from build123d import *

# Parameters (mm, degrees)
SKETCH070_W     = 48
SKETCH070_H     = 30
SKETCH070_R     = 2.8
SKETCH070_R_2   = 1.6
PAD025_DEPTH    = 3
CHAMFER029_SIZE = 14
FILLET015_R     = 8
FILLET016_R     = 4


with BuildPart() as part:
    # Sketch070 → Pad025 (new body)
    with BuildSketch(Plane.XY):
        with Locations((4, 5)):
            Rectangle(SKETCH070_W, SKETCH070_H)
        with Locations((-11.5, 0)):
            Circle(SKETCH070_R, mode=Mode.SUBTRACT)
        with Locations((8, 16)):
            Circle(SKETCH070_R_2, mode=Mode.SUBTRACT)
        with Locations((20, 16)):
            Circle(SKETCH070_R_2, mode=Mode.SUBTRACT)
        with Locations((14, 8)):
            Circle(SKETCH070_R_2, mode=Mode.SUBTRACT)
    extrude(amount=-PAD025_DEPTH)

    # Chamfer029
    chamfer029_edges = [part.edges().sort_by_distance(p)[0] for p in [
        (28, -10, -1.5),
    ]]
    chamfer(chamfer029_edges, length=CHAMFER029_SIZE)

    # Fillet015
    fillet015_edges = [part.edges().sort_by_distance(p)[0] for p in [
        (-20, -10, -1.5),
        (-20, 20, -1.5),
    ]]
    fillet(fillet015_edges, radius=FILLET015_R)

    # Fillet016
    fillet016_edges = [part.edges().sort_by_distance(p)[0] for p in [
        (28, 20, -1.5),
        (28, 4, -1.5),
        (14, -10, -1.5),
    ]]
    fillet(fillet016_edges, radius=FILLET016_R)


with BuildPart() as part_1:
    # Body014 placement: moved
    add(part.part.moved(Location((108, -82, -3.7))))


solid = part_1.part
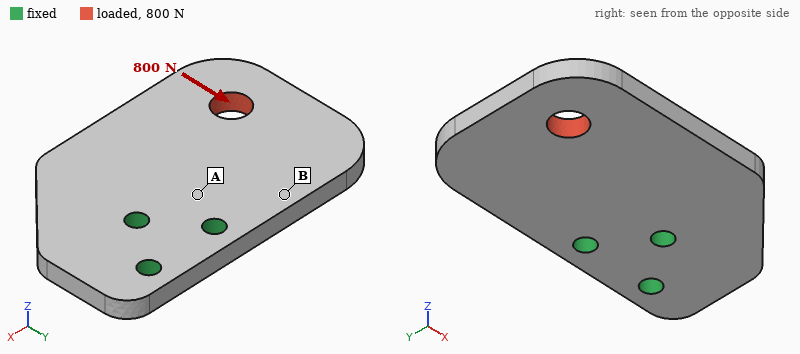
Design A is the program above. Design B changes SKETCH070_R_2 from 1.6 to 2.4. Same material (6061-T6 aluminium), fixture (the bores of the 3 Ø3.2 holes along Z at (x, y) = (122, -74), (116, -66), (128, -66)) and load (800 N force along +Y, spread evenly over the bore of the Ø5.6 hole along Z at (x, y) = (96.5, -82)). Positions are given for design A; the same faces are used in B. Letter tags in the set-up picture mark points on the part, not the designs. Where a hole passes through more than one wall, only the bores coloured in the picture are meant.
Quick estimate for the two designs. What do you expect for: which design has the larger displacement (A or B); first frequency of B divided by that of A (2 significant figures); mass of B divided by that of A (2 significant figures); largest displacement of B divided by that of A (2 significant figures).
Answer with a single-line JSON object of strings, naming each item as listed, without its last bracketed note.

{"which design has the larger displacement": "A", "first frequency of B divided by that of A": "1.1", "mass of B divided by that of A": "0.98", "largest displacement of B divided by that of A": "0.84"}
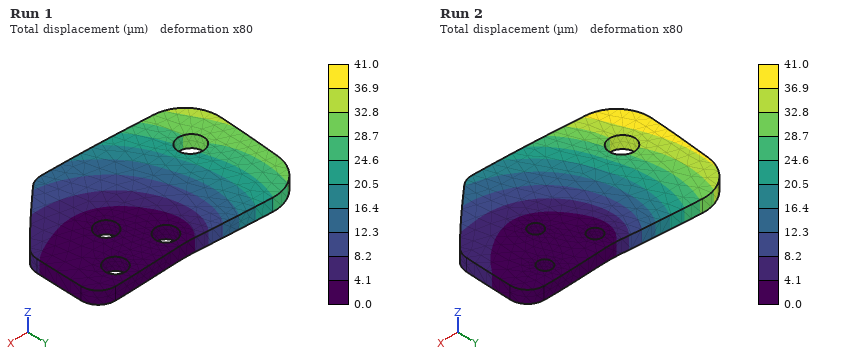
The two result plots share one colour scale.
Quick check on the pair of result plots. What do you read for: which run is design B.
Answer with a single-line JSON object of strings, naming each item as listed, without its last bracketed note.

{"which run is design B": "Run 1"}
